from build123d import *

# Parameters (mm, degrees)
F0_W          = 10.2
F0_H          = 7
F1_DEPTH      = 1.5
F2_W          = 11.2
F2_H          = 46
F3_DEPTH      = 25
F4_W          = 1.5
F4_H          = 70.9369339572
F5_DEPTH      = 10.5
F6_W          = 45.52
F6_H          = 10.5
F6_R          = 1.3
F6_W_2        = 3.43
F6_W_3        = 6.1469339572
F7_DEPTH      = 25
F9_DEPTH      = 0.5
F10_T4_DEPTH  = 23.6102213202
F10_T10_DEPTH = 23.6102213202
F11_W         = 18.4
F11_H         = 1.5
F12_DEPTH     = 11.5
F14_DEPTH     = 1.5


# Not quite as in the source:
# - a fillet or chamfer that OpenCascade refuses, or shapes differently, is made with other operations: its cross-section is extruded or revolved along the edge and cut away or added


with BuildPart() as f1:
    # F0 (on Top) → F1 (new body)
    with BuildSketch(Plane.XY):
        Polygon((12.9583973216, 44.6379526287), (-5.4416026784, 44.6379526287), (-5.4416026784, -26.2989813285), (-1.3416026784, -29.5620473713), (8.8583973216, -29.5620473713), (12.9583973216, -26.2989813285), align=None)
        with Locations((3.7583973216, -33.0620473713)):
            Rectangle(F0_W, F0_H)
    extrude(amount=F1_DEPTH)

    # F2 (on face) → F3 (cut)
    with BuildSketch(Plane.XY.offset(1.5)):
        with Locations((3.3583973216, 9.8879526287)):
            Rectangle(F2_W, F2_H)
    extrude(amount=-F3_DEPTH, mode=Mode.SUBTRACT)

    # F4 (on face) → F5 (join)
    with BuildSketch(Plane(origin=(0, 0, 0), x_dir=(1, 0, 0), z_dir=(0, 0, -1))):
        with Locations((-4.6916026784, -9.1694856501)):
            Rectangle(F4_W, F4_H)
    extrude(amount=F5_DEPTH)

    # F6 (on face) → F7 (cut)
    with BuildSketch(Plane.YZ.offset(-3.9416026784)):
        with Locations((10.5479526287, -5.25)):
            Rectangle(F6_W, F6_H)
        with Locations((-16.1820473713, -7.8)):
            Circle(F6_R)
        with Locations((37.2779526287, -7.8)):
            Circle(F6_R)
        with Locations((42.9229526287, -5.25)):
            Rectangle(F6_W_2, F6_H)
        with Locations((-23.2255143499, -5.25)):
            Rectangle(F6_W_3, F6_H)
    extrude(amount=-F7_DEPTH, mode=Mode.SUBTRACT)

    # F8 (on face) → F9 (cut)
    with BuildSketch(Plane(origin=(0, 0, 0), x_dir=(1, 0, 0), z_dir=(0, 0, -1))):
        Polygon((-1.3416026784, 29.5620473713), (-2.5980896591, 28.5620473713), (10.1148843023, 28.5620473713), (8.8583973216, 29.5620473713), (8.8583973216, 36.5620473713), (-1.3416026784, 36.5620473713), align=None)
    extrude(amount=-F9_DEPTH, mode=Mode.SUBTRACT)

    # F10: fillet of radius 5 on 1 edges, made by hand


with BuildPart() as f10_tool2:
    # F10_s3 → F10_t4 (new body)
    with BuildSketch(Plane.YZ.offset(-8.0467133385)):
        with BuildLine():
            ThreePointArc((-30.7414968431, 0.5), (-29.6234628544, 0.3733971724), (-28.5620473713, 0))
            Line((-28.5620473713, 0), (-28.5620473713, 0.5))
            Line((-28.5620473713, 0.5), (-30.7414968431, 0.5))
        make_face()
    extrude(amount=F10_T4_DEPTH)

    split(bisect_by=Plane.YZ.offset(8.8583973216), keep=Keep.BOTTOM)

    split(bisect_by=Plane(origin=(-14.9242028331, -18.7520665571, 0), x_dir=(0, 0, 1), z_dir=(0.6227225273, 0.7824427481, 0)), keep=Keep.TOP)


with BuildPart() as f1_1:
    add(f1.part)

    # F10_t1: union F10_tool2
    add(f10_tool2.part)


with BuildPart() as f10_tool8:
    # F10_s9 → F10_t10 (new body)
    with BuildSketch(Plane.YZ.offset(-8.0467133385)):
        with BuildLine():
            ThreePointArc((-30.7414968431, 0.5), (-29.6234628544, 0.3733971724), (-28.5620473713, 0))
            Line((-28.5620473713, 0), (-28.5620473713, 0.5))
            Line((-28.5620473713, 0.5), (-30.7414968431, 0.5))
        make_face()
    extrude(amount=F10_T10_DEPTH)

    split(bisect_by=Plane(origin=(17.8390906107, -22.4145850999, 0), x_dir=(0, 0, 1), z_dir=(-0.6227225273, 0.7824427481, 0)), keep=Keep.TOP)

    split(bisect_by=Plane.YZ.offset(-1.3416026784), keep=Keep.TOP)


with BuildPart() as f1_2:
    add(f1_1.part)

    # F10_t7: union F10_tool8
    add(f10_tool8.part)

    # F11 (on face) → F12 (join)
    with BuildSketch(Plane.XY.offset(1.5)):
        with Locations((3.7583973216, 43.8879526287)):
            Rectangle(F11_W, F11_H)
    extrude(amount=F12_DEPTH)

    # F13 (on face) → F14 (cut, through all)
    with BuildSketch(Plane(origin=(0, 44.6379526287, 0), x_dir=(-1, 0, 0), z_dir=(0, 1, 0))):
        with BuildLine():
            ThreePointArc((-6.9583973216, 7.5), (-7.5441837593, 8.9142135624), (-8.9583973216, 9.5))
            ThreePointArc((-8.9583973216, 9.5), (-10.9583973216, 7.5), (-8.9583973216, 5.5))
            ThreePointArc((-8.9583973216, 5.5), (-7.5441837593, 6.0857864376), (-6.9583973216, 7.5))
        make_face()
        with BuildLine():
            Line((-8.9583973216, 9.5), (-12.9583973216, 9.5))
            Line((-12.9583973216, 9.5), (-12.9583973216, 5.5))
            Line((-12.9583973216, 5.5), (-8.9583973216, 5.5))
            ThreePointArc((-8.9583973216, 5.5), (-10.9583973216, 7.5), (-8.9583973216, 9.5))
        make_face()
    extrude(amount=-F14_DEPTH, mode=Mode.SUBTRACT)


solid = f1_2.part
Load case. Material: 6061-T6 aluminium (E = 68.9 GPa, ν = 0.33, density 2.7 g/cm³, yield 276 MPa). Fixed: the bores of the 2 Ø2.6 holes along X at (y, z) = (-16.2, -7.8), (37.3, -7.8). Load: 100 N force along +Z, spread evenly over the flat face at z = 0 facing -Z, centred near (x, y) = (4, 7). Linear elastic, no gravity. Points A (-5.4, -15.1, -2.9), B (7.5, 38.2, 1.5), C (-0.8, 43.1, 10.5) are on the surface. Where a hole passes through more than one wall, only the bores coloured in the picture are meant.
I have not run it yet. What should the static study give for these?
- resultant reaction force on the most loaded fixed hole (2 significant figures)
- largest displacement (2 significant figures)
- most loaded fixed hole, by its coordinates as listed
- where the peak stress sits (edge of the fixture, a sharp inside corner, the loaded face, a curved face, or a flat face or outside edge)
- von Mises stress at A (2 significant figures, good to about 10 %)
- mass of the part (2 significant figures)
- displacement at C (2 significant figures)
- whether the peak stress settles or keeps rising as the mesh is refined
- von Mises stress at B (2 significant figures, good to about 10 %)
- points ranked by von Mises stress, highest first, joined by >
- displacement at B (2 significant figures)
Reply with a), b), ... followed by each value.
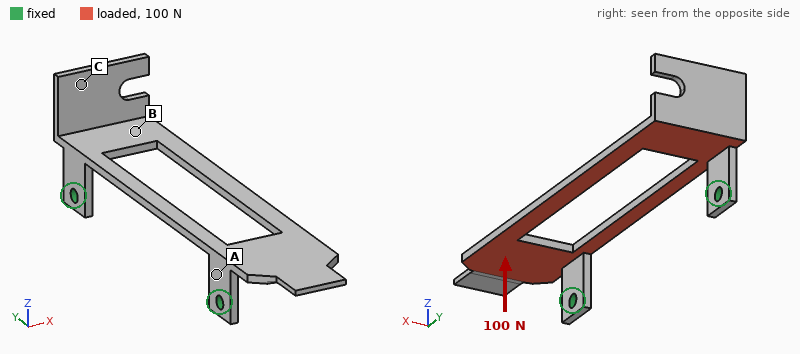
a) 55 N
b) 0.69 mm
c) (-16.2, -7.8)
d) edge of the fixture
e) 140 MPa
f) 5.0 g
g) 0.33 mm
h) keeps rising
i) 33 MPa
j) A > B > C
k) 0.32 mm
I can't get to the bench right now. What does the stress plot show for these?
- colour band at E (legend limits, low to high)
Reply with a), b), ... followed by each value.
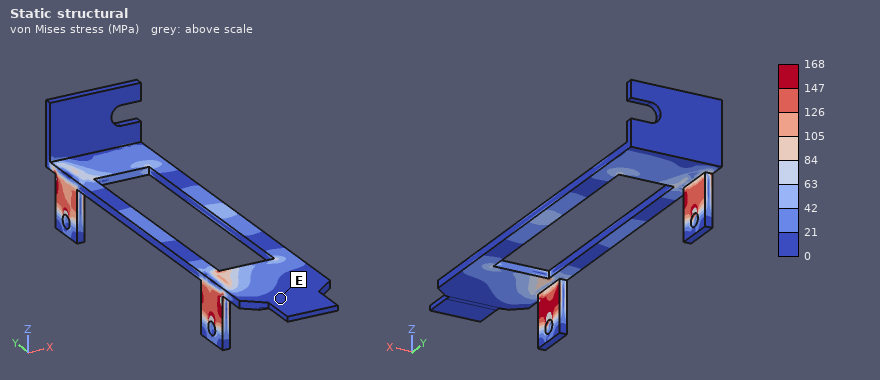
a) 0 to 21 MPa
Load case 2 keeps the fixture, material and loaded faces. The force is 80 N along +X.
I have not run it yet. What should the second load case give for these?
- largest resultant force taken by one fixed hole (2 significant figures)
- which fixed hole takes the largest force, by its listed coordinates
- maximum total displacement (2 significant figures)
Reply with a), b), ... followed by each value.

a) 45 N
b) (-16.2, -7.8)
c) 0.13 mm
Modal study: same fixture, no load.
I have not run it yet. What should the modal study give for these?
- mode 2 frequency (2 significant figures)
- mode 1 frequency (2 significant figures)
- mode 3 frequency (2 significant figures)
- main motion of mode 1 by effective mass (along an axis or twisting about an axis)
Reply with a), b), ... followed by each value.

a) 1500 Hz
b) 1100 Hz
c) 2300 Hz
d) along Z
